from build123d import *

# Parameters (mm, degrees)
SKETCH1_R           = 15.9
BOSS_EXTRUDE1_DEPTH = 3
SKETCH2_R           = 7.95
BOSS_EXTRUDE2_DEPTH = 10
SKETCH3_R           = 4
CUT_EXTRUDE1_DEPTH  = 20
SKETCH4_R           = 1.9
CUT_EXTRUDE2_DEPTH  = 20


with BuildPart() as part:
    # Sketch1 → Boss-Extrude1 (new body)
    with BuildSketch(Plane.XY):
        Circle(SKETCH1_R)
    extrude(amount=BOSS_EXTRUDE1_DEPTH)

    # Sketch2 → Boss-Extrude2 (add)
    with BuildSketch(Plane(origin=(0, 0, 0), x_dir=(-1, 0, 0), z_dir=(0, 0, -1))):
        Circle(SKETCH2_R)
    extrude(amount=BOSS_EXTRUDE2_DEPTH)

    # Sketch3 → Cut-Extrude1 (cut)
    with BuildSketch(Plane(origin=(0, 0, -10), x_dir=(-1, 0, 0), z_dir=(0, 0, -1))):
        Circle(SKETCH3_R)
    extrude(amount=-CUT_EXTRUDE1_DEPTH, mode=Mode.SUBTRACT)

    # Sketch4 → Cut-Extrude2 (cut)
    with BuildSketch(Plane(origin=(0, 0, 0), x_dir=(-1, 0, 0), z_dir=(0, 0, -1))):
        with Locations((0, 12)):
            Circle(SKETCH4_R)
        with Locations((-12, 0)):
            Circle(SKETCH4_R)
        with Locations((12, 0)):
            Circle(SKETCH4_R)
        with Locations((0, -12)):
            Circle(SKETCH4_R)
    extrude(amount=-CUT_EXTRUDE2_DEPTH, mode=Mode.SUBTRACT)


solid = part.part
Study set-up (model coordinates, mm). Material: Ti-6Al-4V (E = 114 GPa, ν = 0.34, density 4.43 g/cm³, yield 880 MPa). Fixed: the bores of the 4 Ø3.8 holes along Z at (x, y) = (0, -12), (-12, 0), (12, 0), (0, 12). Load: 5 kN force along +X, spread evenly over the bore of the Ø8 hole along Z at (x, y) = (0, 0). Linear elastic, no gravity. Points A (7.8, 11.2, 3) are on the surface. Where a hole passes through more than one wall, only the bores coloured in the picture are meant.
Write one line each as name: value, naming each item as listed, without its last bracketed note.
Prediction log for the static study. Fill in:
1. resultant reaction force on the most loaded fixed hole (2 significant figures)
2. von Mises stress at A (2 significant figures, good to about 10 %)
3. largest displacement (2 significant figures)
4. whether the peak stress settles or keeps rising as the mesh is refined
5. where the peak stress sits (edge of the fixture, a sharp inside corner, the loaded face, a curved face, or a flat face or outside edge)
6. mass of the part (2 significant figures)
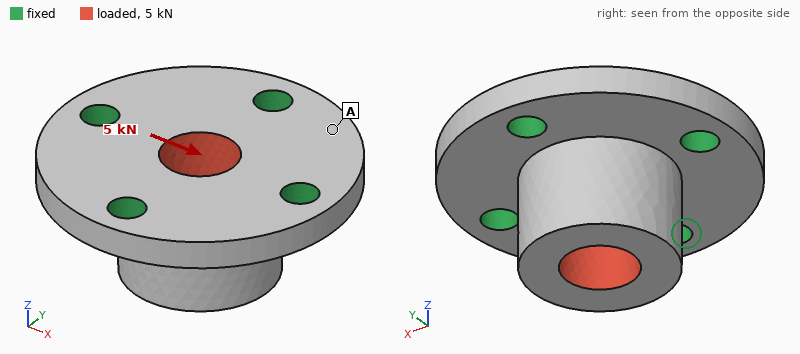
resultant reaction force on the most loaded fixed hole: 2.0 kN
von Mises stress at A: 28 MPa
largest displacement: 20 µm
whether the peak stress settles or keeps rising as the mesh is refined: keeps rising
where the peak stress sits: edge of the fixture
mass of the part: 16 g
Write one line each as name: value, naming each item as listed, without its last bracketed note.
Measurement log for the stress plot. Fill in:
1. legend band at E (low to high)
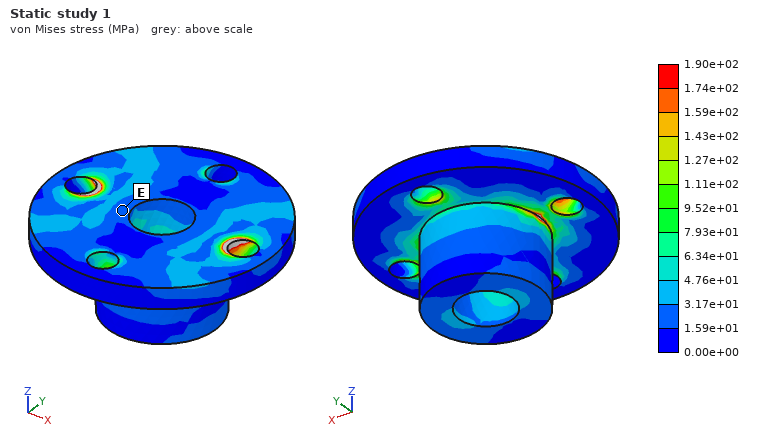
legend band at E: 1.59e+01 to 3.17e+01 MPa
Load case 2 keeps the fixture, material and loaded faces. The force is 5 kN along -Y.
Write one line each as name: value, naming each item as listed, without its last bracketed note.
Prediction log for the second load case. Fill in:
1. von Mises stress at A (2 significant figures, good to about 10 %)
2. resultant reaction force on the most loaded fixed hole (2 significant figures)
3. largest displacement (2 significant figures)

von Mises stress at A: 32 MPa
resultant reaction force on the most loaded fixed hole: 2.0 kN
largest displacement: 20 µm
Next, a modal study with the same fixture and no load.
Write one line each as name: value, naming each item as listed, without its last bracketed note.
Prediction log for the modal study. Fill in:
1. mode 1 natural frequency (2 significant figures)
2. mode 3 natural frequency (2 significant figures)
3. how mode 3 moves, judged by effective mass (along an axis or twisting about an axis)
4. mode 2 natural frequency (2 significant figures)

mode 1 natural frequency: 31 kHz
mode 3 natural frequency: 37 kHz
how mode 3 moves, judged by effective mass: along Z
mode 2 natural frequency: 31 kHz
